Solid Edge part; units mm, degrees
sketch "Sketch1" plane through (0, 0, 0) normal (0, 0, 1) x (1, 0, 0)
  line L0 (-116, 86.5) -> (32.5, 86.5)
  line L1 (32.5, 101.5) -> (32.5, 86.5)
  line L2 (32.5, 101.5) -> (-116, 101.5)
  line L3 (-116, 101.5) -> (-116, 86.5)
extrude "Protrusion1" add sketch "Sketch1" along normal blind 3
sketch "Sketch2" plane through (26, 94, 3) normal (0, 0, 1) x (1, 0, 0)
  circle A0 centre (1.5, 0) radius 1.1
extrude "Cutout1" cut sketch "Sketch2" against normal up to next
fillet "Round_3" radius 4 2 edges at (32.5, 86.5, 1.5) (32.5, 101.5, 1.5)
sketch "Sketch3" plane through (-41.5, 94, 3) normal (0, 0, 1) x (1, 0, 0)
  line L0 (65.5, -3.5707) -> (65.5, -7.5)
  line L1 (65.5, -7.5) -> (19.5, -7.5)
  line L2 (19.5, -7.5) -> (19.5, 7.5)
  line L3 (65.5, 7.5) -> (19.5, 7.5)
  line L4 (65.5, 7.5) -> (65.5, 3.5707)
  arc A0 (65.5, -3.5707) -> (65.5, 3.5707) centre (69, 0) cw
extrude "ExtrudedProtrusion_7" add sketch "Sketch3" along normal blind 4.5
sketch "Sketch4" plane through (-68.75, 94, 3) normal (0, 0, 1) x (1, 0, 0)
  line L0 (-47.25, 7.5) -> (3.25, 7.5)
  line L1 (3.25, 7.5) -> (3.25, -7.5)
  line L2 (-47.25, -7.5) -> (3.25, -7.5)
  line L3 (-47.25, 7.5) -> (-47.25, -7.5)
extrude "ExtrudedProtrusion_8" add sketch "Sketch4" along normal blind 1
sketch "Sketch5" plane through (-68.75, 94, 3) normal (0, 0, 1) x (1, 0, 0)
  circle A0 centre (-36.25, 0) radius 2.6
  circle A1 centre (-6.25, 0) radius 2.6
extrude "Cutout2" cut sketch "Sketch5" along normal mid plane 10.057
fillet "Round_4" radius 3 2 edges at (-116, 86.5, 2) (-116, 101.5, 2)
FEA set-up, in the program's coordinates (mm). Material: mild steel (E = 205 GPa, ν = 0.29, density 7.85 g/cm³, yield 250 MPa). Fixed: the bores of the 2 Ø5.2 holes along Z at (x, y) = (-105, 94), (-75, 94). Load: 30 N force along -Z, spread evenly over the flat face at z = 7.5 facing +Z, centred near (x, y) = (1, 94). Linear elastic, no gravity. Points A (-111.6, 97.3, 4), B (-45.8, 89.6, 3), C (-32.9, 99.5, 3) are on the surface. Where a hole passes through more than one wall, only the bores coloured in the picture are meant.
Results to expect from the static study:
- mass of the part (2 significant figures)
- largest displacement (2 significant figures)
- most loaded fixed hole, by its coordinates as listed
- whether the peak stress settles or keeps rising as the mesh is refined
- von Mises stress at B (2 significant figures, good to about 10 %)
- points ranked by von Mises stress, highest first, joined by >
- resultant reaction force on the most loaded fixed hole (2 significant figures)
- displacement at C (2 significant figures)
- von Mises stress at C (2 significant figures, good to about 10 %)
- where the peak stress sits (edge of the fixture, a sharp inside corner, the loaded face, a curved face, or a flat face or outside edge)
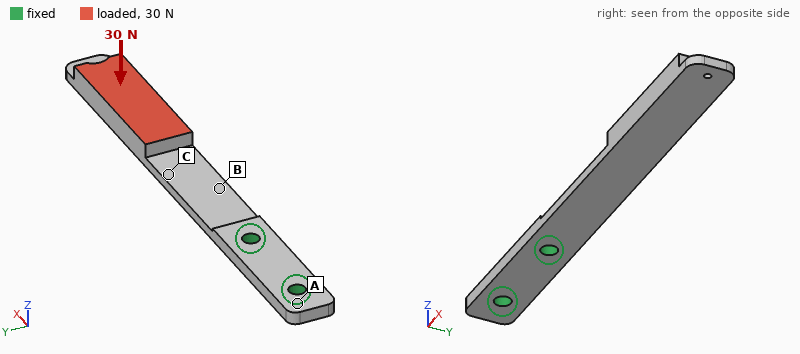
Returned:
81 g
0.79 mm
(-75, 94)
keeps rising
62 MPa
B > C > A
32 N
0.17 mm
45 MPa
edge of the fixture
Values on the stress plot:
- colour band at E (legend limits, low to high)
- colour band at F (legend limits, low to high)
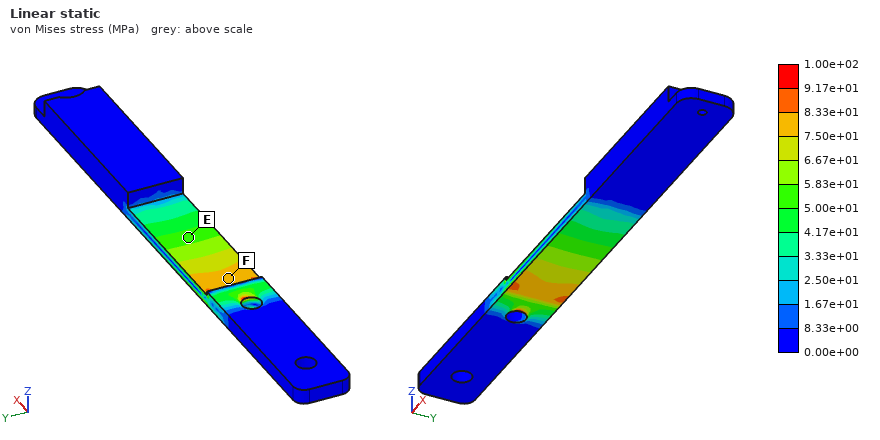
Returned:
5.00e+01 to 5.83e+01 MPa
7.50e+01 to 8.33e+01 MPa
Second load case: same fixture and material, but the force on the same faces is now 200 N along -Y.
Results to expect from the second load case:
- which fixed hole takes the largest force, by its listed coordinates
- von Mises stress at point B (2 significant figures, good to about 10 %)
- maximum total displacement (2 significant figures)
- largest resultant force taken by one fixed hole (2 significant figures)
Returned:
(-75, 94)
76 MPa
0.30 mm
410 N
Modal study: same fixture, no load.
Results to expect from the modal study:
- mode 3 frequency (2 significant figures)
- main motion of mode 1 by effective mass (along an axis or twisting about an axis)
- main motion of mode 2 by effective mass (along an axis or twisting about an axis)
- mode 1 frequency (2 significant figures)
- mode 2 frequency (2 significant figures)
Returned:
1600 Hz
along Z
along Y
170 Hz
740 Hz
